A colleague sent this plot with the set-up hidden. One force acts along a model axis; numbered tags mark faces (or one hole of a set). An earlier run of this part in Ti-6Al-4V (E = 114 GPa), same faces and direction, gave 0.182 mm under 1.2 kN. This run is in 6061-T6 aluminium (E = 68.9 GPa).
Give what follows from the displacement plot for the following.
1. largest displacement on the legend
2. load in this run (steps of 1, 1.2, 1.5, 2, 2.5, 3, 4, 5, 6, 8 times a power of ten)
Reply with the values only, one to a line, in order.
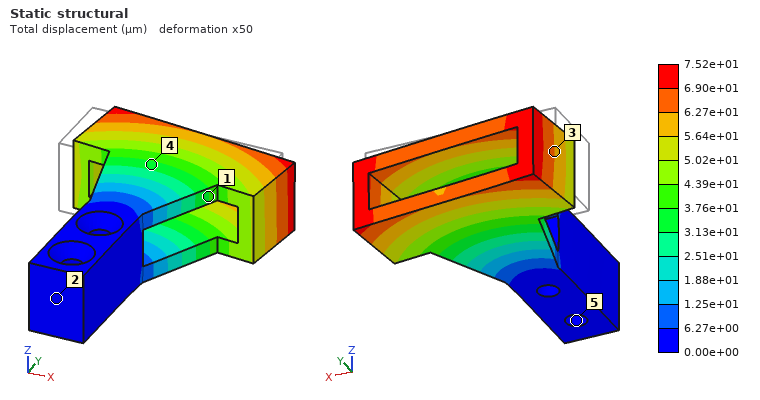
7.52e+01 µm
300 N
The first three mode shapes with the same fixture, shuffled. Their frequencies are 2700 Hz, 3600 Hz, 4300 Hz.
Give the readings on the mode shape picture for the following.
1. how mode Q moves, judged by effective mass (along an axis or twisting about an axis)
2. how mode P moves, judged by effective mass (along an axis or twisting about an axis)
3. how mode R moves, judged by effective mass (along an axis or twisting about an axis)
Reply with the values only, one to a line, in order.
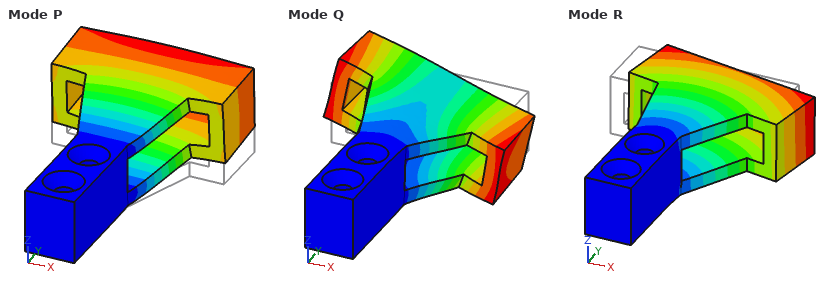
twisting about Y
along Z
along X
